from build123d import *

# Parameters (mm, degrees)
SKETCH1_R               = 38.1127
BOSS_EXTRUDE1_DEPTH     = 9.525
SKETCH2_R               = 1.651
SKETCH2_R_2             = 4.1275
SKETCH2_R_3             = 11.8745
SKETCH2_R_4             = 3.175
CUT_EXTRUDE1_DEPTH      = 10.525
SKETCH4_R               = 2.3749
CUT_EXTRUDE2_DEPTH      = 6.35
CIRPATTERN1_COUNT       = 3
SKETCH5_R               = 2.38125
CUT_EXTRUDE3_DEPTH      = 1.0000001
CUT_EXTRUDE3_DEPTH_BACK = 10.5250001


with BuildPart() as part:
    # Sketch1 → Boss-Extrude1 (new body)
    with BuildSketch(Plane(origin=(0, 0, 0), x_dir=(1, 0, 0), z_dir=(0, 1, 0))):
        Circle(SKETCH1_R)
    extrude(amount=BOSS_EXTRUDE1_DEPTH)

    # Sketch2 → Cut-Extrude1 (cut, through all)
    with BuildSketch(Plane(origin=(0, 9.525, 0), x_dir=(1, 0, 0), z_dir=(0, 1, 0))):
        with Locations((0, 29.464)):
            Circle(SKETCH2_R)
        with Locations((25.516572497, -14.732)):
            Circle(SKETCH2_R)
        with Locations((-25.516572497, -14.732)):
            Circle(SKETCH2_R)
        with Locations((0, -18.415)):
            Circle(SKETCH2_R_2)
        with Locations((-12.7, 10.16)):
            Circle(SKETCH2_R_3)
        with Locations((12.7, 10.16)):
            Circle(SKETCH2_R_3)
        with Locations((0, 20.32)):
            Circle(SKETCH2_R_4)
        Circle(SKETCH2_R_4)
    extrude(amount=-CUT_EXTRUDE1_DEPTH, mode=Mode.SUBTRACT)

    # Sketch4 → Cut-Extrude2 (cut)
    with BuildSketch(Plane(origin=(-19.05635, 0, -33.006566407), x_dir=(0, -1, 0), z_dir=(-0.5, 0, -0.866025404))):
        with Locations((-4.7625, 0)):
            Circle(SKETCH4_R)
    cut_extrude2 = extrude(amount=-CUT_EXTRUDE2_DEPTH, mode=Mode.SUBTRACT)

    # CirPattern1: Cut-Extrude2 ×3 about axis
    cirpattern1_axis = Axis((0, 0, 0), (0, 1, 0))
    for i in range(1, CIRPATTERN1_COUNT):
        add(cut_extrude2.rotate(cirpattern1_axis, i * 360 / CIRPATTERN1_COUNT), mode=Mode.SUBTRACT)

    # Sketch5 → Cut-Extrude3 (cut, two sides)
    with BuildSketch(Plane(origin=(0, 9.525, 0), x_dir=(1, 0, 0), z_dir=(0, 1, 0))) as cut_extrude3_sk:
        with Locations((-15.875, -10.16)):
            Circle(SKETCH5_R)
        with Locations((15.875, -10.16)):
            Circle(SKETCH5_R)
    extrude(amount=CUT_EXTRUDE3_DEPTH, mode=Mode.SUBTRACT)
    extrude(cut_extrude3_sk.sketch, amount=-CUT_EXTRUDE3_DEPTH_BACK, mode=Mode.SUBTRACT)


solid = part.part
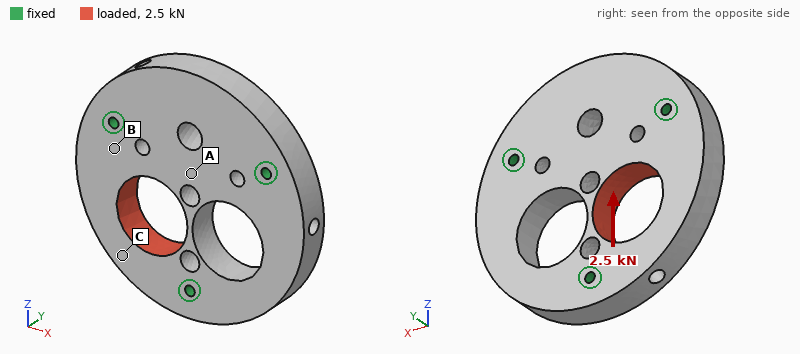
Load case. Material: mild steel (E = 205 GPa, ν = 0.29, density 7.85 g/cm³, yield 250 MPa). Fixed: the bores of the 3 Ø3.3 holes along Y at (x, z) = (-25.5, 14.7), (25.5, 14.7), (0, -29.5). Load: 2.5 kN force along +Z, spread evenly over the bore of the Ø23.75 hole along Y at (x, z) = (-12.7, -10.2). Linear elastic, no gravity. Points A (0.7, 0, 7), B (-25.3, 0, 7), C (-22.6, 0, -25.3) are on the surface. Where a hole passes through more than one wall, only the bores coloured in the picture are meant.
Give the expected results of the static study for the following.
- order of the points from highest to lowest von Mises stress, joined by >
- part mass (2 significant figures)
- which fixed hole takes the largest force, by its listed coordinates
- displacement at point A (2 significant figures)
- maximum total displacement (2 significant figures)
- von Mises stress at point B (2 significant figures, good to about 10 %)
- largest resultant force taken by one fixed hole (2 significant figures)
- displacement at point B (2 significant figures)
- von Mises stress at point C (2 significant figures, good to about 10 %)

B > C > A
260 g
(-25.5, 14.7)
0.63 µm
1.7 µm
9.6 MPa
1.5 kN
0.40 µm
5.2 MPa
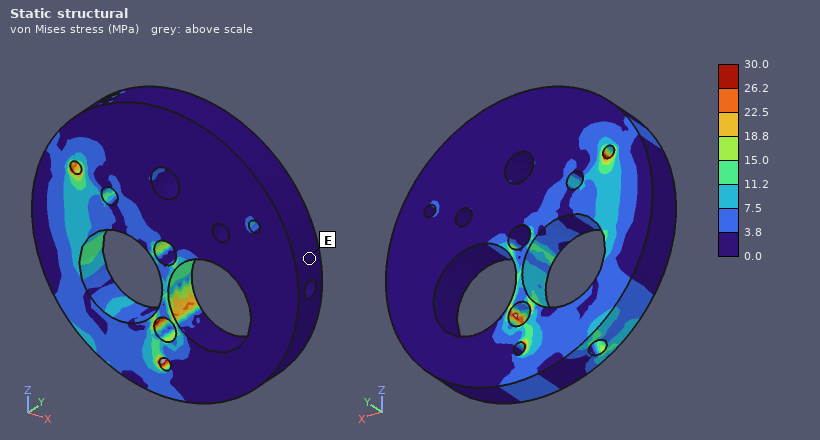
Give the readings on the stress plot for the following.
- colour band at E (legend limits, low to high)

0.0 to 3.8 MPa
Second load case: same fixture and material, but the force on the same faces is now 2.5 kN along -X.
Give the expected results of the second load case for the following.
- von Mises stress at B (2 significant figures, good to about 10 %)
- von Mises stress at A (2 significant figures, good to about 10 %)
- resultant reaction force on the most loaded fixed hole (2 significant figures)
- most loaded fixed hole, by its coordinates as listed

4.9 MPa
4.6 MPa
1.3 kN
(0, -29.5)
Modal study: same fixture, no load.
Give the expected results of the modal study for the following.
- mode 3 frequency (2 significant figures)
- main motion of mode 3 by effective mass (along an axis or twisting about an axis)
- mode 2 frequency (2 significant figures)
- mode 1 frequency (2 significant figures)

10 kHz
along Y
9000 Hz
8700 Hz
